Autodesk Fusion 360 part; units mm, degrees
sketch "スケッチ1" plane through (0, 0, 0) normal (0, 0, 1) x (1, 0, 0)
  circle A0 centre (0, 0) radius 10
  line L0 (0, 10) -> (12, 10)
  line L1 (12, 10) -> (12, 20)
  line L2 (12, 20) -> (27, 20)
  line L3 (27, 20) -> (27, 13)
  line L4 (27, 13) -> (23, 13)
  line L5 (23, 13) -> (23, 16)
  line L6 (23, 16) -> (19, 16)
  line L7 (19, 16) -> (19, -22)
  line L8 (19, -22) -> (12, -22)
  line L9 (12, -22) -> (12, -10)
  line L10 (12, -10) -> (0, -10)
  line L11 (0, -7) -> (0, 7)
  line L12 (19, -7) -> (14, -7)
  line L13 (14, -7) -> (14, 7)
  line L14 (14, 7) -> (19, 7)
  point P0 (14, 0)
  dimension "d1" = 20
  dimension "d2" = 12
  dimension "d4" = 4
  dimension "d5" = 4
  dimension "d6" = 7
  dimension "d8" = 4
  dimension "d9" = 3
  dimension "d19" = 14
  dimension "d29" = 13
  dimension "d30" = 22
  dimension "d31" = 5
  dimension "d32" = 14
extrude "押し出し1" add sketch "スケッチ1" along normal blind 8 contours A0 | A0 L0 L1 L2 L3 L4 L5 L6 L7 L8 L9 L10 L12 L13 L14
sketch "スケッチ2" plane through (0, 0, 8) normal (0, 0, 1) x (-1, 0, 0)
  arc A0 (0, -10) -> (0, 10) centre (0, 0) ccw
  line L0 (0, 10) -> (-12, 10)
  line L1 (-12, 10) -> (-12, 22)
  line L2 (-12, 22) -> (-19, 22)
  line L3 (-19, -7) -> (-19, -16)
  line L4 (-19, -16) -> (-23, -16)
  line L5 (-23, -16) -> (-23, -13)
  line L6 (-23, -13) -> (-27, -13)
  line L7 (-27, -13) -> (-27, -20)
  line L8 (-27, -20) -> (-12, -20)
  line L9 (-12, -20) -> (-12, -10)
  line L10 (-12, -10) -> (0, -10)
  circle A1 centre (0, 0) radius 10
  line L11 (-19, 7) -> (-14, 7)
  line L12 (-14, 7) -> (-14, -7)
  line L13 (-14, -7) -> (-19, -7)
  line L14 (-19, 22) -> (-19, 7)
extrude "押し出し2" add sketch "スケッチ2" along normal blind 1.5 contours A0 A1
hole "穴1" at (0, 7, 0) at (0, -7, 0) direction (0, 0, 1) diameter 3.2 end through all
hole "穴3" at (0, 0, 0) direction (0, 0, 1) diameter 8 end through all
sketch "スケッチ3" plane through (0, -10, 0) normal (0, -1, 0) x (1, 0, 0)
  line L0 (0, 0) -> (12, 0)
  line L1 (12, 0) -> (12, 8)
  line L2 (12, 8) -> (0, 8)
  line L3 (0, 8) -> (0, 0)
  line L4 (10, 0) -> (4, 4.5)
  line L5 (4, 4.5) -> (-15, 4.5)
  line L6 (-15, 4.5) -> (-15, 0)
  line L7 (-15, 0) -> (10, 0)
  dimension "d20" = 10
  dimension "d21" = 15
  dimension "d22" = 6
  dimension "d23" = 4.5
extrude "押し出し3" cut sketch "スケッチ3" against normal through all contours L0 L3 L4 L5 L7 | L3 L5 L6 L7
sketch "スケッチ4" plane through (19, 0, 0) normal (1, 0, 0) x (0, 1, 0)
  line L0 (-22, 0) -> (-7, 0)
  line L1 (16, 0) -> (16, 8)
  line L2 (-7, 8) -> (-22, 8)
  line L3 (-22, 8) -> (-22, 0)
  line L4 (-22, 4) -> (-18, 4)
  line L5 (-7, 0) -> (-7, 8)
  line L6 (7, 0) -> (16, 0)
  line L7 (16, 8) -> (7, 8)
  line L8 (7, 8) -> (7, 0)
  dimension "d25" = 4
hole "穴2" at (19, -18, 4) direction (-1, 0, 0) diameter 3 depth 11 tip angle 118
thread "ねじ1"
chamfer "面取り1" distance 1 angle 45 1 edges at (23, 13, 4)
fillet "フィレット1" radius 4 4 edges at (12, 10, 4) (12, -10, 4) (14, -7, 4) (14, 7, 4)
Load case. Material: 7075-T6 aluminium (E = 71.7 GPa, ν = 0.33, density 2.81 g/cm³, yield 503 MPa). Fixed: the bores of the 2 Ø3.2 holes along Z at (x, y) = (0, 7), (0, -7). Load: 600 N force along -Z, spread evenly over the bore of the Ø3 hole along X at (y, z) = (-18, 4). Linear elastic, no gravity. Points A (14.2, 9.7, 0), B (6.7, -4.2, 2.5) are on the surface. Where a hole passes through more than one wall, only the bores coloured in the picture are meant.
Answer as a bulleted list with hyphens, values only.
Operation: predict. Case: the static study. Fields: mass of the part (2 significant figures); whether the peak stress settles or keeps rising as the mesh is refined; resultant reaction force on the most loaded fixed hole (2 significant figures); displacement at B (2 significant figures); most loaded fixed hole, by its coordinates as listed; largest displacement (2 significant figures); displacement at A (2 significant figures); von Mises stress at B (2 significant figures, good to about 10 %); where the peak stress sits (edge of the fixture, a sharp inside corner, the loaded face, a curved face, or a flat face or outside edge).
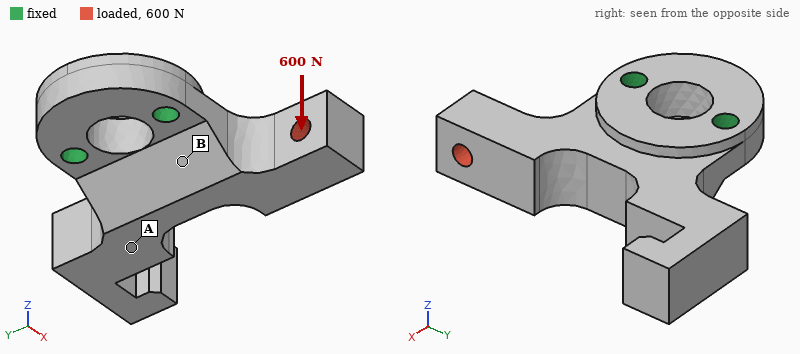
- 12 g
- keeps rising
- 950 N
- 0.032 mm
- (0, -7)
- 0.20 mm
- 0.032 mm
- 85 MPa
- edge of the fixture
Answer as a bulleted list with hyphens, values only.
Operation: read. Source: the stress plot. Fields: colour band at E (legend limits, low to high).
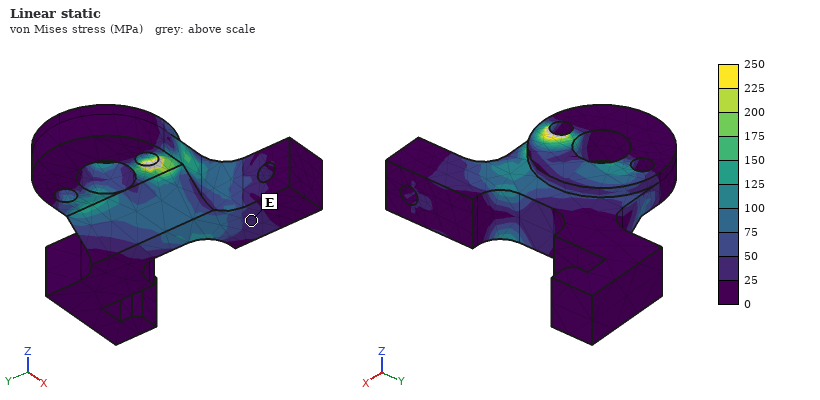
- 25 to 50 MPa
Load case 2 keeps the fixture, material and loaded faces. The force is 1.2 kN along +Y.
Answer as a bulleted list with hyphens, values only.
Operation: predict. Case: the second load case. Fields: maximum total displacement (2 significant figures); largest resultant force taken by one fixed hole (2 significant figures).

- 52 µm
- 1.4 kN
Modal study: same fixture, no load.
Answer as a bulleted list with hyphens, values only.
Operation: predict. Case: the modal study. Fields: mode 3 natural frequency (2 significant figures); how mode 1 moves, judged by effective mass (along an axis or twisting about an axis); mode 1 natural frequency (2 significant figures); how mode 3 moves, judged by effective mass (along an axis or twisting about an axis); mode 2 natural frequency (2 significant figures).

- 9700 Hz
- along Z
- 4900 Hz
- along Y
- 7600 Hz
